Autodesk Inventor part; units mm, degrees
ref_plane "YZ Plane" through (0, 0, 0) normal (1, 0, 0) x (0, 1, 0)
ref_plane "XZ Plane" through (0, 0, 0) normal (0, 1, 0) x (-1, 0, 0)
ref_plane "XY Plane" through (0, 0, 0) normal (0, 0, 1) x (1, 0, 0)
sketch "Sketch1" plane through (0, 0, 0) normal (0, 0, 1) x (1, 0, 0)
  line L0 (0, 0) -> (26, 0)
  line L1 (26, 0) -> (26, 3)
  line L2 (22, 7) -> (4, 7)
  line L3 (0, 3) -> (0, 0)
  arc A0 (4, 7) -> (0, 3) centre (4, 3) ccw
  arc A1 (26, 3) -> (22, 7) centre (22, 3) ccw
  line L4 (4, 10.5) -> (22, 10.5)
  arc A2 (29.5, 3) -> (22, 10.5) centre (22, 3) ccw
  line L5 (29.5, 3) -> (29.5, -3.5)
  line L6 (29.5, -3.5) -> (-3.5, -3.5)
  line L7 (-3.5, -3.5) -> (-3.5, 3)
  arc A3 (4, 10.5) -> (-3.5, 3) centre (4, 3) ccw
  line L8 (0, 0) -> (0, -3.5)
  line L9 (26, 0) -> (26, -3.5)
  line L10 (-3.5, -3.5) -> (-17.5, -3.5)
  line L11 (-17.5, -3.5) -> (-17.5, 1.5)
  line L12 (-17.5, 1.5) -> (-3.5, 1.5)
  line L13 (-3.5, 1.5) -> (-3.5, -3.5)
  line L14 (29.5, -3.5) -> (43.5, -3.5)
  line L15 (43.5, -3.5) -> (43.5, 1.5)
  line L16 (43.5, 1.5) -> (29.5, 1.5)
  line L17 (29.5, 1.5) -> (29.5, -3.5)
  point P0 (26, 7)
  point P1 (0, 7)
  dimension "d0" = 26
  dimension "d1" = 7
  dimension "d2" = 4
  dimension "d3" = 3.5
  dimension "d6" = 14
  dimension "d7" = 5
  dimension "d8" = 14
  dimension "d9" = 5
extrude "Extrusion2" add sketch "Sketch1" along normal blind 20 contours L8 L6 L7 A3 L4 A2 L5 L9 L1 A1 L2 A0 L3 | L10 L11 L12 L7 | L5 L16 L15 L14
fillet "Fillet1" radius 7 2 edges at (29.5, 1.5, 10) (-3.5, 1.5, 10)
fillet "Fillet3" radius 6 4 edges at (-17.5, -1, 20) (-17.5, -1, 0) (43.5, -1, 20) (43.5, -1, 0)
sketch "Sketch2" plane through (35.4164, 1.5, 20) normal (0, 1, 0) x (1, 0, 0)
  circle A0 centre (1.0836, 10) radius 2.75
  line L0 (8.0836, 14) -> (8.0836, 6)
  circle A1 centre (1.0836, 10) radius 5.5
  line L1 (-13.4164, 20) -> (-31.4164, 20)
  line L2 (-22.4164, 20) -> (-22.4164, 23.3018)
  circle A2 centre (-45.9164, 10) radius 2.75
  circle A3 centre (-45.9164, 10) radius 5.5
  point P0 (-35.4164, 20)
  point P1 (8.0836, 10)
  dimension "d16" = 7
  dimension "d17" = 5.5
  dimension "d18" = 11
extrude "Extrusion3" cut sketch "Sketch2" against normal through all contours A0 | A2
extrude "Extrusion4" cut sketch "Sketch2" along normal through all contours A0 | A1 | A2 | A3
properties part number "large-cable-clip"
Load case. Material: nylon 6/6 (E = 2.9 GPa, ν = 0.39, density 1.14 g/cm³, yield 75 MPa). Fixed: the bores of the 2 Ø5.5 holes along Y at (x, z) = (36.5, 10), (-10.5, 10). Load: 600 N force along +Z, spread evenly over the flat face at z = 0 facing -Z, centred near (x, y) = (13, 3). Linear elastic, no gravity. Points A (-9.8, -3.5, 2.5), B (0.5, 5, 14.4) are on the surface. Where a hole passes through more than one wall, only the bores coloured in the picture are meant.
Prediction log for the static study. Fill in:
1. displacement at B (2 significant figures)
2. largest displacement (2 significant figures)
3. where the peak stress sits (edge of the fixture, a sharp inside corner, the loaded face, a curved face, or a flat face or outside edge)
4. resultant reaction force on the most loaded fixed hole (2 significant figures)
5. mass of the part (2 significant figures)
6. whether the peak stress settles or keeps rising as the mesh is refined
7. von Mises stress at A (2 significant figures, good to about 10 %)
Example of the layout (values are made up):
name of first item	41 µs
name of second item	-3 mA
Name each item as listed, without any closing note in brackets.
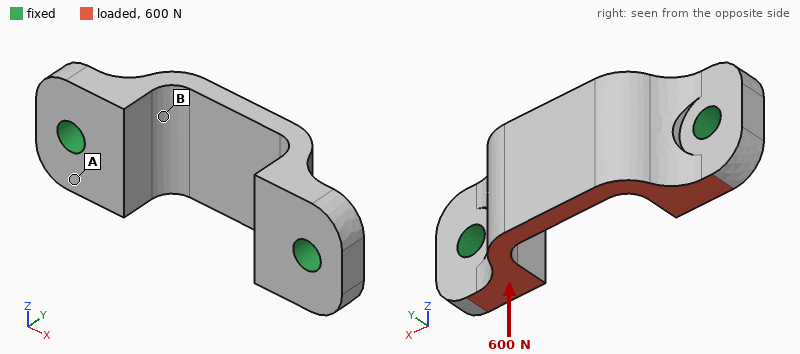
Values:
displacement at B	0.11 mm
largest displacement	0.22 mm
where the peak stress sits	edge of the fixture
resultant reaction force on the most loaded fixed hole	300 N
mass of the part	6.9 g
whether the peak stress settles or keeps rising as the mesh is refined	keeps rising
von Mises stress at A	6.8 MPa
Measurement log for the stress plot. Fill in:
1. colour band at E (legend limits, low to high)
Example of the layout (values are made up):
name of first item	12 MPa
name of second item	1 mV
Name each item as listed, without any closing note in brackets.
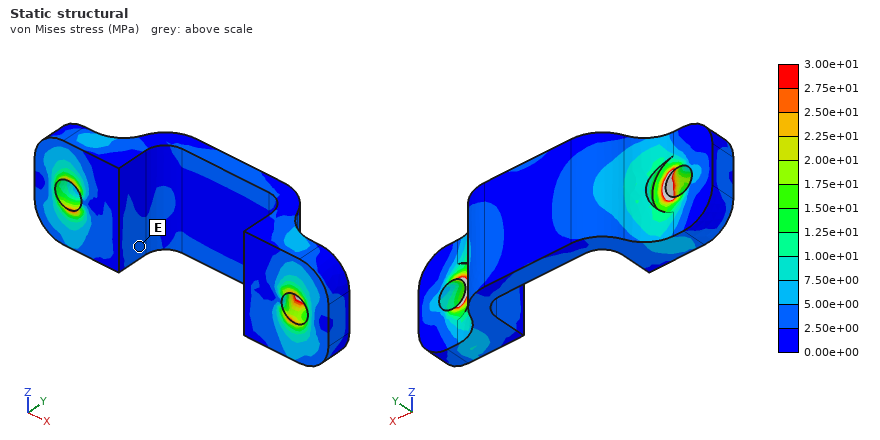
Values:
colour band at E	2.50e+00 to 5.00e+00 MPa
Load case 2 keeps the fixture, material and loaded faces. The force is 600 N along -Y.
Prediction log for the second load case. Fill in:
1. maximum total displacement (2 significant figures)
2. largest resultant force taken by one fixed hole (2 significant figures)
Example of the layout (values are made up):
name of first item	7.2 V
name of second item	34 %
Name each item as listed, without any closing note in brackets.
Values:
maximum total displacement	0.50 mm
largest resultant force taken by one fixed hole	340 N
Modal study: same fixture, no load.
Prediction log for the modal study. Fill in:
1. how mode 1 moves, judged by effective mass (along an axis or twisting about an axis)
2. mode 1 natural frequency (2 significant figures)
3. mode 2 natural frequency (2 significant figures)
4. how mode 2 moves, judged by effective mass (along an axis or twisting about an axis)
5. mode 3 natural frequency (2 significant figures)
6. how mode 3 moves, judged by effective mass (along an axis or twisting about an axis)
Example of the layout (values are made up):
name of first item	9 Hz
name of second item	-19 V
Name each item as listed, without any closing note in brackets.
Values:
how mode 1 moves, judged by effective mass	along Z
mode 1 natural frequency	3900 Hz
mode 2 natural frequency	5100 Hz
how mode 2 moves, judged by effective mass	along X
mode 3 natural frequency	6100 Hz
how mode 3 moves, judged by effective mass	along Y
